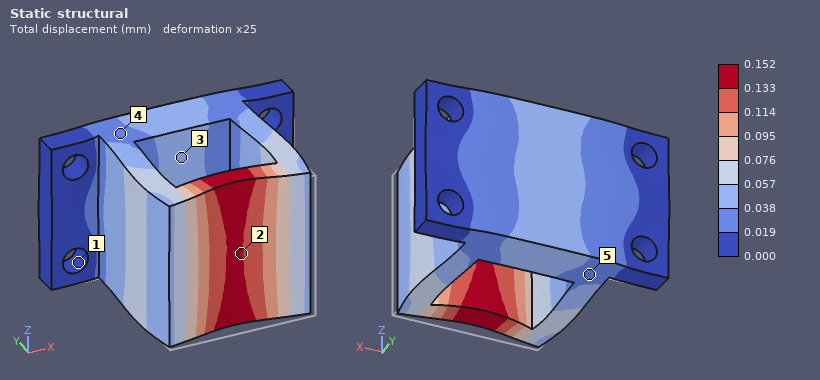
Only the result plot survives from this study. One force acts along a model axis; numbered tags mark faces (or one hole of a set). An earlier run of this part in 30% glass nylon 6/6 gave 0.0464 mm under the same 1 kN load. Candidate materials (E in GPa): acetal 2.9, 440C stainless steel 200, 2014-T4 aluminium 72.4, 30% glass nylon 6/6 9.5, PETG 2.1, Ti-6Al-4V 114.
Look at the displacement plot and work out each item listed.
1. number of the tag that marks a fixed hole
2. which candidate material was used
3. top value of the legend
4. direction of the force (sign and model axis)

1
acetal
0.152 mm
+Y
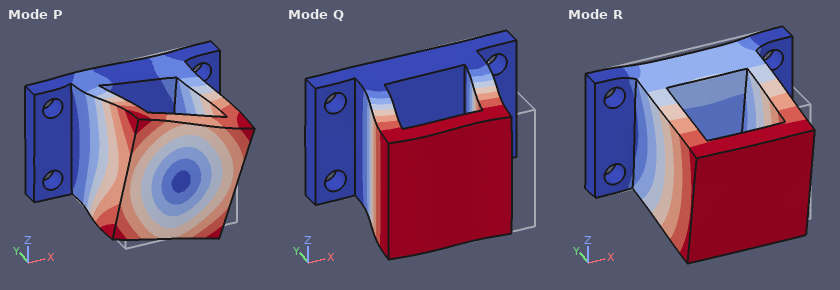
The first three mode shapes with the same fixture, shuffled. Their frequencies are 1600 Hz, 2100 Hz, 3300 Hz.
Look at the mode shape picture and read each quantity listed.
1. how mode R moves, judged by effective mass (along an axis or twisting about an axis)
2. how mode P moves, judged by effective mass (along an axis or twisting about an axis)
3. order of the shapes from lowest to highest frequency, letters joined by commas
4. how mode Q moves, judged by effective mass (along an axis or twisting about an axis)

along Z
twisting about Y
Q, R, P
along X
